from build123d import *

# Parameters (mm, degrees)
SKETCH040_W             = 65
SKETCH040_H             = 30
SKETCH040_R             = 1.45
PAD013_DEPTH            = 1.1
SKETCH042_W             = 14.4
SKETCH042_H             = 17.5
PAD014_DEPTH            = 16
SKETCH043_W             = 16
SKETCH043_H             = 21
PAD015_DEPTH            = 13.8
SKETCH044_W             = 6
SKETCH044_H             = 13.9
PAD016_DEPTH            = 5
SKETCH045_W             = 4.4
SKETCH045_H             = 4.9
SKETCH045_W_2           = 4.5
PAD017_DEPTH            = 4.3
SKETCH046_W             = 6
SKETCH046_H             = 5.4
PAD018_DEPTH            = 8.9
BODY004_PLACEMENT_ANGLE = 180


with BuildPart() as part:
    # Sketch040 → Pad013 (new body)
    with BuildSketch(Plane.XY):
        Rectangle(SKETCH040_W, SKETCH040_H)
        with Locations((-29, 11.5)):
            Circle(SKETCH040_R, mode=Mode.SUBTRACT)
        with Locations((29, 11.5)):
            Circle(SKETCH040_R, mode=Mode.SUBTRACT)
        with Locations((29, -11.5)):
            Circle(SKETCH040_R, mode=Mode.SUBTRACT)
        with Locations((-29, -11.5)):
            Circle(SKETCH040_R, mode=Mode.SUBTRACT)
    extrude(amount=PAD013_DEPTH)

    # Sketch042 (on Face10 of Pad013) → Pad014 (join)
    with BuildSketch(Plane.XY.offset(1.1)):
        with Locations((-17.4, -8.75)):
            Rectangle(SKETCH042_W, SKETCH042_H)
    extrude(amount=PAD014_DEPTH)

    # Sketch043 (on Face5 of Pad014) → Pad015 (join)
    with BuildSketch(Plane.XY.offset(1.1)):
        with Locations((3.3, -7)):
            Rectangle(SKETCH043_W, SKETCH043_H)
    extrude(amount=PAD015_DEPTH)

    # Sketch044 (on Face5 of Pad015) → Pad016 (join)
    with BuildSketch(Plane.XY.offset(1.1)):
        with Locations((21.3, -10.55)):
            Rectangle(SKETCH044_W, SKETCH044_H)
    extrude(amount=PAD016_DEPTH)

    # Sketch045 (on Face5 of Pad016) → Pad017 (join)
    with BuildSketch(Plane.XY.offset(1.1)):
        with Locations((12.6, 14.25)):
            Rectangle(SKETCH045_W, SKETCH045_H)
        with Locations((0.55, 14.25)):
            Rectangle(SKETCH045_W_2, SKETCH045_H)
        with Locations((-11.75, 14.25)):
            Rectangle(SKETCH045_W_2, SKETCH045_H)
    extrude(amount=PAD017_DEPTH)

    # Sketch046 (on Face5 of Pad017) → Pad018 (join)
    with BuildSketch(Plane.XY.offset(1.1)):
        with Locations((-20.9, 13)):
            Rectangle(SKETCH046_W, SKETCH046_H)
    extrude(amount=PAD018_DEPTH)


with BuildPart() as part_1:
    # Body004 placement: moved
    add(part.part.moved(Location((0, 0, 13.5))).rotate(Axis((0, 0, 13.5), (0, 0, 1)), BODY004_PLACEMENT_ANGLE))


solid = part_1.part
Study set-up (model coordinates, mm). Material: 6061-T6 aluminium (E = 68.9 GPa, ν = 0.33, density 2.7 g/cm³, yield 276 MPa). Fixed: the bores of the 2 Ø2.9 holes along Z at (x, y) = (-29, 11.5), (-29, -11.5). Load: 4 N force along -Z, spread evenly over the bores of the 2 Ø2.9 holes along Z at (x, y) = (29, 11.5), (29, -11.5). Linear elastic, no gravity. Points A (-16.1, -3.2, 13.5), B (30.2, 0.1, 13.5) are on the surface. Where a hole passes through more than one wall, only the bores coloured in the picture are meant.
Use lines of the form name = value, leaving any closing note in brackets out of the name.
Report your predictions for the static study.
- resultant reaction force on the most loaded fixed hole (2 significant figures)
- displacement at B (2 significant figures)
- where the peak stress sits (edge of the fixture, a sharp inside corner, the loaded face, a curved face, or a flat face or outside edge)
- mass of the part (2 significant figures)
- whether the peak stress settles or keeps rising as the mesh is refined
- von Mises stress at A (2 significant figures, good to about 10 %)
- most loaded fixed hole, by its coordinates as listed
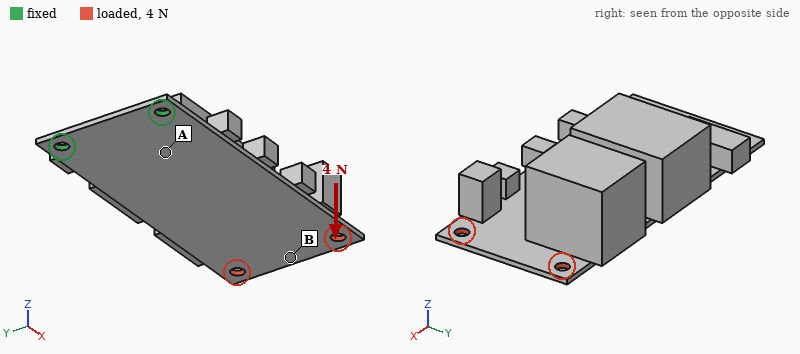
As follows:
resultant reaction force on the most loaded fixed hole = 2.8 N
displacement at B = 0.71 mm
where the peak stress sits = edge of the fixture
mass of the part = 32 g
whether the peak stress settles or keeps rising as the mesh is refined = keeps rising
von Mises stress at A = 23 MPa
most loaded fixed hole, by its coordinates as listed = (-29, -11.5)
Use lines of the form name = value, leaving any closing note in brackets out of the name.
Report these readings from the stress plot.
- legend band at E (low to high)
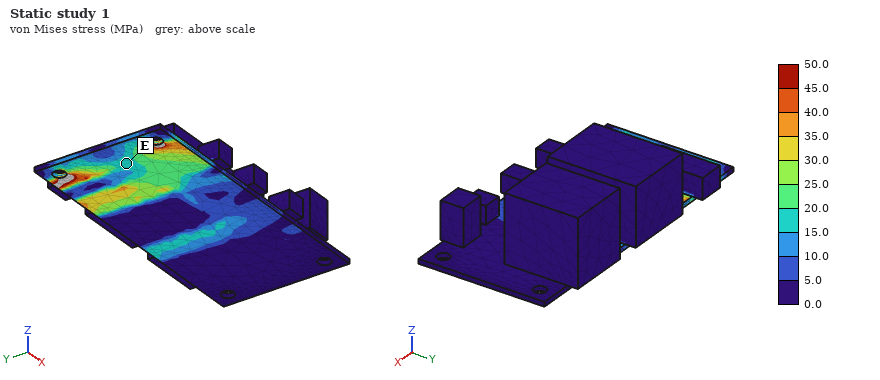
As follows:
legend band at E = 15.0 to 20.0 MPa
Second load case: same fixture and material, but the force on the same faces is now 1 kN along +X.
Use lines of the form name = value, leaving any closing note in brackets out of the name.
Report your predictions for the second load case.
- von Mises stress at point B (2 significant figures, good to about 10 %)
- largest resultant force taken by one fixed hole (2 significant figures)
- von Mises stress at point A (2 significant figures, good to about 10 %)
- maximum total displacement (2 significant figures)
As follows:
von Mises stress at point B = 17 MPa
largest resultant force taken by one fixed hole = 510 N
von Mises stress at point A = 26 MPa
maximum total displacement = 0.12 mm
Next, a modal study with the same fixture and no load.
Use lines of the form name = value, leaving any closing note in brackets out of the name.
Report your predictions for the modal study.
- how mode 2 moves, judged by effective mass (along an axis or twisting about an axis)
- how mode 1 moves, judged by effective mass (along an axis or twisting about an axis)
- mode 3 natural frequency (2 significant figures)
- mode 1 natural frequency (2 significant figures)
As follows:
how mode 2 moves, judged by effective mass = along Y
how mode 1 moves, judged by effective mass = along Z
mode 3 natural frequency = 770 Hz
mode 1 natural frequency = 120 Hz
